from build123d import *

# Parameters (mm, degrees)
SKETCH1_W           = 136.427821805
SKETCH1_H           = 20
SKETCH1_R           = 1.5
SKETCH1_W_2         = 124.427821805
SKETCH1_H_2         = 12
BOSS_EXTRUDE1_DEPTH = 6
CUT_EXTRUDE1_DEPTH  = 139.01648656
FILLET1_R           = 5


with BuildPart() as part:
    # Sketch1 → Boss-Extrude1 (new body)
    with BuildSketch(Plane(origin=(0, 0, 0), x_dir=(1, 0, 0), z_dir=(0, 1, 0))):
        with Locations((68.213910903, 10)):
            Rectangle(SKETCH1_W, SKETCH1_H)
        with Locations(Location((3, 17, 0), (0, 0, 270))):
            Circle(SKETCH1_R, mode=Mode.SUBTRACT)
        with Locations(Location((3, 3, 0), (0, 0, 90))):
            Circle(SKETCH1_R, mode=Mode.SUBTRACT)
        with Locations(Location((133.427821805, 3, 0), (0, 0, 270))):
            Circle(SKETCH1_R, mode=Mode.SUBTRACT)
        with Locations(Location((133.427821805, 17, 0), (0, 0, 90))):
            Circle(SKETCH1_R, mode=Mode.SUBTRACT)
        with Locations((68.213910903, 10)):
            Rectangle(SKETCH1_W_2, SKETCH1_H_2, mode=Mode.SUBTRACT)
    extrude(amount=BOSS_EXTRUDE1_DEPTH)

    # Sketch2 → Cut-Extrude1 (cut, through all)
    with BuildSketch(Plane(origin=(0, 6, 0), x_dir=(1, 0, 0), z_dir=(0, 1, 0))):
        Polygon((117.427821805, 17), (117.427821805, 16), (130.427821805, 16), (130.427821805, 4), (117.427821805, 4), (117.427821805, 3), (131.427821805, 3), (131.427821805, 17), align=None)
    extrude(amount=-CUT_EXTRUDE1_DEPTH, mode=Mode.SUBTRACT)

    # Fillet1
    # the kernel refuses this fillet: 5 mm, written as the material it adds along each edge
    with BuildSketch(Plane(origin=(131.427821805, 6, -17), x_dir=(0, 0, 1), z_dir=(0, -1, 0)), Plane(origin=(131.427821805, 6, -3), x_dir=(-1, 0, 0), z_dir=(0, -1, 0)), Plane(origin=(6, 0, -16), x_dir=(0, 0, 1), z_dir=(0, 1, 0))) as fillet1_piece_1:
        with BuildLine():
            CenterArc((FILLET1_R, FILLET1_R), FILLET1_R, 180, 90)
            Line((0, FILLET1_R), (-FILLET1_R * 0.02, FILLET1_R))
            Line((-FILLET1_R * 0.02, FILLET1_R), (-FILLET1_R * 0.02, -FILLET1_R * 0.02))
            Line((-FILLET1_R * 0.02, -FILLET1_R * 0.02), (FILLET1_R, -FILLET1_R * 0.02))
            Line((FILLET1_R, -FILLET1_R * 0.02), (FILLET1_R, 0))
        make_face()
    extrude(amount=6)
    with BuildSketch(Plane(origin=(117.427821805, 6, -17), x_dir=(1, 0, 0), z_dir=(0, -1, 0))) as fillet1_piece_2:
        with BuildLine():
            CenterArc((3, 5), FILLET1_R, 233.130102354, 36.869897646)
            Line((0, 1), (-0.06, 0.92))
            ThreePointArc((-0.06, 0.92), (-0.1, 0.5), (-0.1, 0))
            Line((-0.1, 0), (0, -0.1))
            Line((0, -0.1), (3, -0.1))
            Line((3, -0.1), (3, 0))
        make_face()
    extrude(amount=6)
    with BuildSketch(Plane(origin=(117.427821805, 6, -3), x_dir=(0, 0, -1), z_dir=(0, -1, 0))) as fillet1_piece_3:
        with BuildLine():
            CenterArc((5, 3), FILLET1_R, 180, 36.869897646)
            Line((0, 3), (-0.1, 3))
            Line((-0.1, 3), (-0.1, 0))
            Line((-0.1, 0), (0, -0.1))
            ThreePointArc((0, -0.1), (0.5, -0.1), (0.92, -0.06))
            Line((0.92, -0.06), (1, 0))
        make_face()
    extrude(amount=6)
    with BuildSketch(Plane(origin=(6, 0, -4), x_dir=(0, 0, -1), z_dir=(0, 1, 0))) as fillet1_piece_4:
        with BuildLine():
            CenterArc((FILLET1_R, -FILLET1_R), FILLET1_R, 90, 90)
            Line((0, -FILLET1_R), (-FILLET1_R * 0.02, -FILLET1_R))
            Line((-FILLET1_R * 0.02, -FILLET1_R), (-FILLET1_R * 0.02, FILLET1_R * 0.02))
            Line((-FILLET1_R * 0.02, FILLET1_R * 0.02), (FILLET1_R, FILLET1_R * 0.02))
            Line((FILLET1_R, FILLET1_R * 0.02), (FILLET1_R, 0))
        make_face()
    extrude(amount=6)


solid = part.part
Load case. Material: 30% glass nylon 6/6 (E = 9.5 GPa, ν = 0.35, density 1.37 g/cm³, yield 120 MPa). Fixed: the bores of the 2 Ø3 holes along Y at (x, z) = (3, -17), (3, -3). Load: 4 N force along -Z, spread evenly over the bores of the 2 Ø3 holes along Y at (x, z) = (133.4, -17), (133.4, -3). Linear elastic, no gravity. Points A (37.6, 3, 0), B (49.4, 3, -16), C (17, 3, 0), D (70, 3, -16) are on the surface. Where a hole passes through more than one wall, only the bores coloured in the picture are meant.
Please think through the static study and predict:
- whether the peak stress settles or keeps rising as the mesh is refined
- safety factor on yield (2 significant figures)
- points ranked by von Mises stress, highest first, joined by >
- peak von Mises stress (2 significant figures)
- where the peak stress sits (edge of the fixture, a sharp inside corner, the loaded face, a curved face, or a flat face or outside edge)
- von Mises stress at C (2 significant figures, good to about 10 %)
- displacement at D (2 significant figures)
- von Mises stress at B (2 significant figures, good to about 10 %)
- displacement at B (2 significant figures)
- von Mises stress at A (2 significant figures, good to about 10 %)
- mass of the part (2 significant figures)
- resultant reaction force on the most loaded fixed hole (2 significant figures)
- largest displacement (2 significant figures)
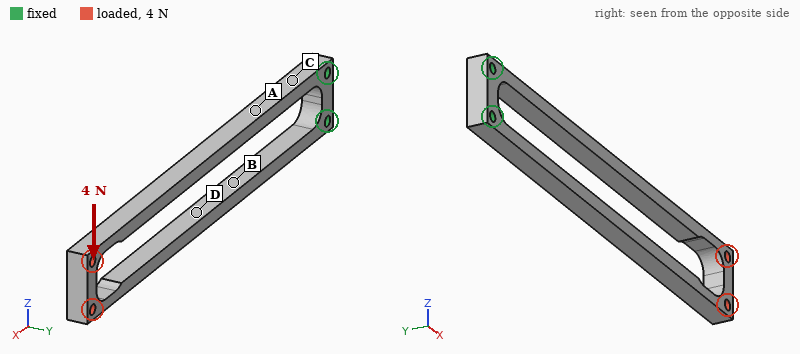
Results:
settles
9.0
C > A > B > D
13 MPa
a curved face
8.2 MPa
0.66 mm
2.9 MPa
0.34 mm
5.6 MPa
9.8 g
26 N
1.5 mm
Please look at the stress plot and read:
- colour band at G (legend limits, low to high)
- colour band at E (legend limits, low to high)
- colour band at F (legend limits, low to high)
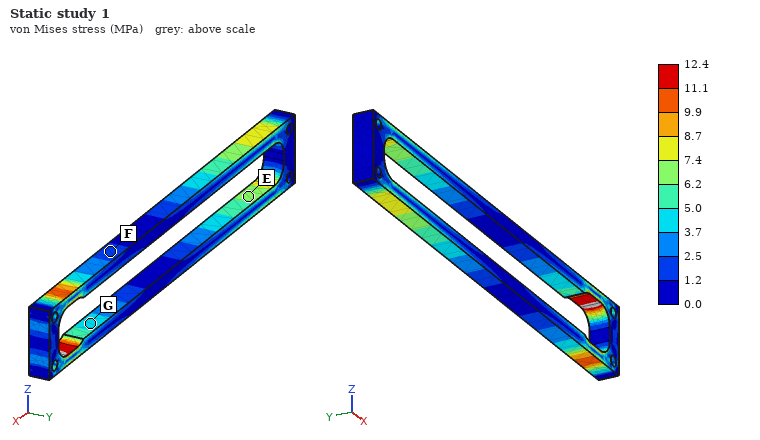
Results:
3.7 to 5.0 MPa
6.2 to 7.4 MPa
1.2 to 2.5 MPa
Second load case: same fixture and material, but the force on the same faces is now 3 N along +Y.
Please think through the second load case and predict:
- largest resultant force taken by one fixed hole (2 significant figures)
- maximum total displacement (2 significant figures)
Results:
1.5 N
1.6 mm
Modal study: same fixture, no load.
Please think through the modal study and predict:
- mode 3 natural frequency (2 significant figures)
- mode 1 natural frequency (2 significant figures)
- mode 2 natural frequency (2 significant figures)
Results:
610 Hz
140 Hz
140 Hz
